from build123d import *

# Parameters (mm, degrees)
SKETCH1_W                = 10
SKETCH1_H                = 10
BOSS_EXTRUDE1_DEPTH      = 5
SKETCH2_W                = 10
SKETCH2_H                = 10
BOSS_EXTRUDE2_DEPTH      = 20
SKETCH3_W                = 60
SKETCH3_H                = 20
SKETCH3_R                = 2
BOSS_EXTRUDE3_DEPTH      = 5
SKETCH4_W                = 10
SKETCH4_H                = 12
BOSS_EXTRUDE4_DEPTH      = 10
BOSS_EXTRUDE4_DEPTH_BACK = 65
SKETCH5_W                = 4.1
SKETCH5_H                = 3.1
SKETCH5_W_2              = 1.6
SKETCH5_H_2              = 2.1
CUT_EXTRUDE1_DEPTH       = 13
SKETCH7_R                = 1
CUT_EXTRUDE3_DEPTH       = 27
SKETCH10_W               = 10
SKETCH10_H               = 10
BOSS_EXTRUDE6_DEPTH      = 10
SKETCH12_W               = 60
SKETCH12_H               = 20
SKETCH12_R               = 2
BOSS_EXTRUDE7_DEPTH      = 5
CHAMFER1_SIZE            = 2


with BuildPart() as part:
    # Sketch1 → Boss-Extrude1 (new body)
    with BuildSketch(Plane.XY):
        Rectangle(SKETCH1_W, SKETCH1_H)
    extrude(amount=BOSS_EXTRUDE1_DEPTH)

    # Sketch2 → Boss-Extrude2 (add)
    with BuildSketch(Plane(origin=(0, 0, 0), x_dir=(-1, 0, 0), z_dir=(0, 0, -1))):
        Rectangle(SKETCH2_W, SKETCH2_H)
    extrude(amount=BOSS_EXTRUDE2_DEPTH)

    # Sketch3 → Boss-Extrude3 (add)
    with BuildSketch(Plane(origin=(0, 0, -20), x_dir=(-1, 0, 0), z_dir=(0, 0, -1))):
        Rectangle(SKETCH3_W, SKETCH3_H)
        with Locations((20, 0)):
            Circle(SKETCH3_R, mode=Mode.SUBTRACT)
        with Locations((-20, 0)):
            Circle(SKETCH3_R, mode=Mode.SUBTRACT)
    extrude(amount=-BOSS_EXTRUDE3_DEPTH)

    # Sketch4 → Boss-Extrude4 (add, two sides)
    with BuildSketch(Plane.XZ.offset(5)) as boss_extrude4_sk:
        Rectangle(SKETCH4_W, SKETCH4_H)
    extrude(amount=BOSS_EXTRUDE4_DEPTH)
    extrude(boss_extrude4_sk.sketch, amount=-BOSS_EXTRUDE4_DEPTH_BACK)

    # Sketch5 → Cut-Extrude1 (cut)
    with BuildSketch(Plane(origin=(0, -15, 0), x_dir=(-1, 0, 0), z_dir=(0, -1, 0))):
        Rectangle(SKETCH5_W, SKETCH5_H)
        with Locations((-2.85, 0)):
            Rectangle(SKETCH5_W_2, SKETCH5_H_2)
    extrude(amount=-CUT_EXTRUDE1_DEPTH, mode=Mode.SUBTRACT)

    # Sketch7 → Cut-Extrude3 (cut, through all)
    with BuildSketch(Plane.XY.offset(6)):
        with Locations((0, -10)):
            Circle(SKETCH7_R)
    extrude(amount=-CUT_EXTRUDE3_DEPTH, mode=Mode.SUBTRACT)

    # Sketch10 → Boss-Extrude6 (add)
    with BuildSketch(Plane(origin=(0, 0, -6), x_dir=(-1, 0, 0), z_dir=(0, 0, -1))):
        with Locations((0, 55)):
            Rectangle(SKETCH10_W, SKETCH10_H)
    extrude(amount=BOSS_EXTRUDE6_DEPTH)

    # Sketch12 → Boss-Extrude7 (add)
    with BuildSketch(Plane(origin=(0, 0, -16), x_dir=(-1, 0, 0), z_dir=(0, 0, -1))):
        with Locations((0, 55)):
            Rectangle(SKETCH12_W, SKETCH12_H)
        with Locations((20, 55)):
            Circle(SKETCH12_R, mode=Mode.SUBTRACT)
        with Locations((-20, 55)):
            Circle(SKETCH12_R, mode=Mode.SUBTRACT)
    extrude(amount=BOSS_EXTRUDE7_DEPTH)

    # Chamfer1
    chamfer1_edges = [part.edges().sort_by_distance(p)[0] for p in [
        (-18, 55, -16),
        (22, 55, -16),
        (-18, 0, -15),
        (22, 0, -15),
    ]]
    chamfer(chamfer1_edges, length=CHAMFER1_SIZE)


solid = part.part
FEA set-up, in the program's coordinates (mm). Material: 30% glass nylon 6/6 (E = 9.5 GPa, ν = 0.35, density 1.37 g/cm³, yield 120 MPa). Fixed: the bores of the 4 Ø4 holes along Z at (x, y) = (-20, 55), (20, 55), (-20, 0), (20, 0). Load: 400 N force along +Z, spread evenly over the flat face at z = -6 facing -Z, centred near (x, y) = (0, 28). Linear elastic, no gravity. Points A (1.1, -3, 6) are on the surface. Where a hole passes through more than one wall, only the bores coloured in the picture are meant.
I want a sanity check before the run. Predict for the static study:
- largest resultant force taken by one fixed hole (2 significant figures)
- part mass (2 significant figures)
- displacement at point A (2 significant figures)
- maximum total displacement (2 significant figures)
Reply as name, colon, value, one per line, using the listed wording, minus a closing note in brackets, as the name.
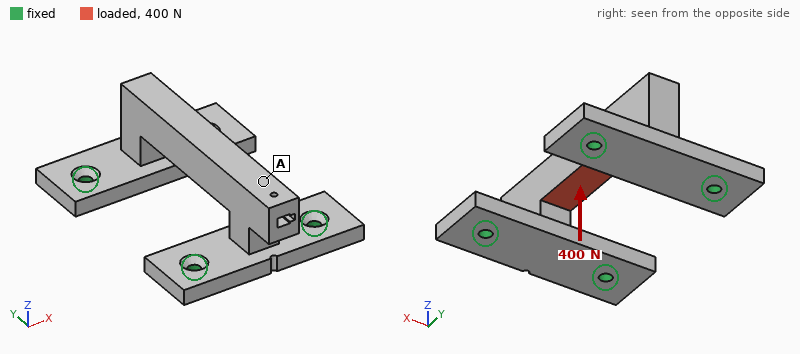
largest resultant force taken by one fixed hole: 140 N
part mass: 31 g
displacement at point A: 38 µm
maximum total displacement: 74 µm
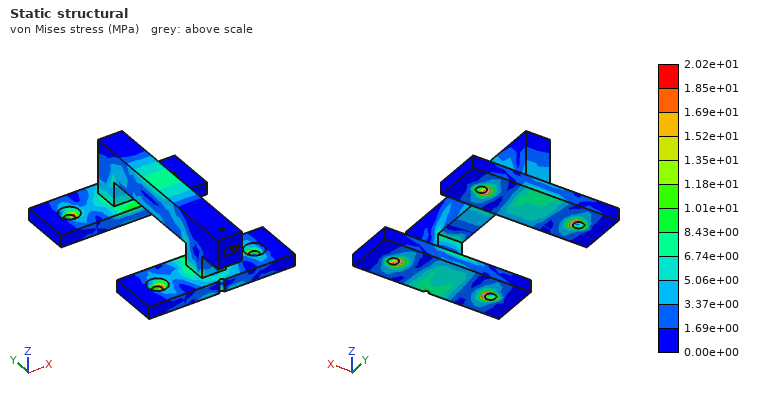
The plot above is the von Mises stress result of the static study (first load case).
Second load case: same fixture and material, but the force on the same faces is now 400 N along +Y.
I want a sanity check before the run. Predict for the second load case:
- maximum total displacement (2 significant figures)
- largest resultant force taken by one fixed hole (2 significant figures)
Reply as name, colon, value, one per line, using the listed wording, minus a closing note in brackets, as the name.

maximum total displacement: 95 µm
largest resultant force taken by one fixed hole: 110 N
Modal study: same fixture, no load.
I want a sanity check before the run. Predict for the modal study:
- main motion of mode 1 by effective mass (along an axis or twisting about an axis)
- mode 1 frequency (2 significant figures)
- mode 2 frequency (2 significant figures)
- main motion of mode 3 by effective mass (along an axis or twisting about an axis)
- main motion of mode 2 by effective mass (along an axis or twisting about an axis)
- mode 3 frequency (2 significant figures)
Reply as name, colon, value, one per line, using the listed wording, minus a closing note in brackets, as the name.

main motion of mode 1 by effective mass: along X
mode 1 frequency: 2600 Hz
mode 2 frequency: 2900 Hz
main motion of mode 3 by effective mass: along Z
main motion of mode 2 by effective mass: along Y
mode 3 frequency: 3400 Hz
